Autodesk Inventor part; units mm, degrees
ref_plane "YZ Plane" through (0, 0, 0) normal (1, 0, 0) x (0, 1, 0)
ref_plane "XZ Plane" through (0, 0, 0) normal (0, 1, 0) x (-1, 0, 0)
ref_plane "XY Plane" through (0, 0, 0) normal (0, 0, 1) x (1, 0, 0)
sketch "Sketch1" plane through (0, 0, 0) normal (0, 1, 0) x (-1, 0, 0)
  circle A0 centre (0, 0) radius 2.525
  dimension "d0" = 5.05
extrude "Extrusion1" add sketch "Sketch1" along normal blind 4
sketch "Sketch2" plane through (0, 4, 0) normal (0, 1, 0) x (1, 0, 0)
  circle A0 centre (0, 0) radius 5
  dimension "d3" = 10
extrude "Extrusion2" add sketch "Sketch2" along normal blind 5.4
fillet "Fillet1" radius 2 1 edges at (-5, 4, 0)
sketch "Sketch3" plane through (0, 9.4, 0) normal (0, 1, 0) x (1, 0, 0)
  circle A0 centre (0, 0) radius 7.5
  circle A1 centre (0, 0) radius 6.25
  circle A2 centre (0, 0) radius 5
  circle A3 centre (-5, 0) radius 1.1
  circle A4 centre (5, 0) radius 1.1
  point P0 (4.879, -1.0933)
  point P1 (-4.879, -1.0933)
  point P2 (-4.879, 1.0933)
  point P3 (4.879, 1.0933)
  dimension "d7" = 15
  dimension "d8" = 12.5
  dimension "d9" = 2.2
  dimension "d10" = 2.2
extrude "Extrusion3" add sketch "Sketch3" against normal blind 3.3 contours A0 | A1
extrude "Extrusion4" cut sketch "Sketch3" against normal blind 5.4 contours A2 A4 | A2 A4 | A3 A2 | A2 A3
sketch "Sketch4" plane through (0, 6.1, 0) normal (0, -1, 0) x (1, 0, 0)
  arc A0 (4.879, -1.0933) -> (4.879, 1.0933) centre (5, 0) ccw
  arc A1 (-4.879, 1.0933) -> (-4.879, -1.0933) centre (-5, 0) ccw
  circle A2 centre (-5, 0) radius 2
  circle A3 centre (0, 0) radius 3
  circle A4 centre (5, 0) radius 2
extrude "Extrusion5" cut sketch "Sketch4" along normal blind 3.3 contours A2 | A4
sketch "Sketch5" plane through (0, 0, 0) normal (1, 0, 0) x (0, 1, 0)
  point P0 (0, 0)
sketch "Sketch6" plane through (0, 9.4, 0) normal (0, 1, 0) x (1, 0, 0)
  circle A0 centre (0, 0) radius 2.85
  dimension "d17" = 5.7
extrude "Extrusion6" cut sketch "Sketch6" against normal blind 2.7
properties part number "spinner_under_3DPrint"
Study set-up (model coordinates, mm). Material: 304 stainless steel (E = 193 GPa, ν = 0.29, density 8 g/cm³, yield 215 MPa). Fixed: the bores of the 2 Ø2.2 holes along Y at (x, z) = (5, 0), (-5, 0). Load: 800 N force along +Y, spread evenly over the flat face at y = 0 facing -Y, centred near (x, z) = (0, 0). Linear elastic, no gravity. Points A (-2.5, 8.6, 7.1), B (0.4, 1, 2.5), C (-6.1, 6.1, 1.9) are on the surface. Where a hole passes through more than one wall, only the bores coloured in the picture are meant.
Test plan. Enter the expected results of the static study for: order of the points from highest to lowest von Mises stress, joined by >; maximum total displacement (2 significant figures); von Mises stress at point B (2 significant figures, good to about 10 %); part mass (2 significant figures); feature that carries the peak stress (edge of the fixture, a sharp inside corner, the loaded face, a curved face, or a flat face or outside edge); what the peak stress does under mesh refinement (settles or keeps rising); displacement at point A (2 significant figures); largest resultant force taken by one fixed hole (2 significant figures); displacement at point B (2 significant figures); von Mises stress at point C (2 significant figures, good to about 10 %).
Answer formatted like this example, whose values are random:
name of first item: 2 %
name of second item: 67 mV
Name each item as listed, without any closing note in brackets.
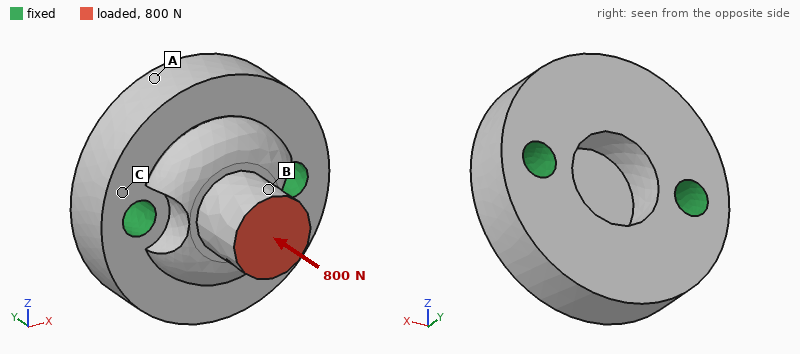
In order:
order of the points from highest to lowest von Mises stress, joined by >: B > C > A
maximum total displacement: 2.2 µm
von Mises stress at point B: 39 MPa
part mass: 5.5 g
feature that carries the peak stress: edge of the fixture
what the peak stress does under mesh refinement: keeps rising
displacement at point A: 1.1 µm
largest resultant force taken by one fixed hole: 430 N
displacement at point B: 2.0 µm
von Mises stress at point C: 14 MPa
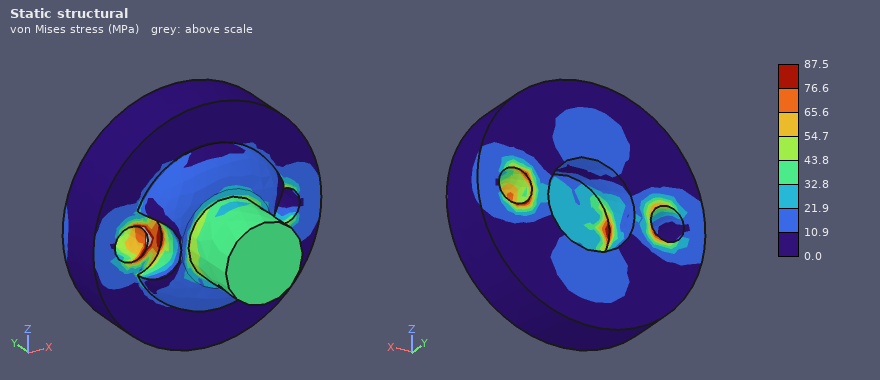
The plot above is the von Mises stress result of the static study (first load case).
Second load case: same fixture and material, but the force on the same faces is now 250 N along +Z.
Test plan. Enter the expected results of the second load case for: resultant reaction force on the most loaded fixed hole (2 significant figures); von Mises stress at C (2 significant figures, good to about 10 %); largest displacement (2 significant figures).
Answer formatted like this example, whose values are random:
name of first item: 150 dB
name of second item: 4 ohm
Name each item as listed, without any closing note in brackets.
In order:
resultant reaction force on the most loaded fixed hole: 130 N
von Mises stress at C: 25 MPa
largest displacement: 5.8 µm
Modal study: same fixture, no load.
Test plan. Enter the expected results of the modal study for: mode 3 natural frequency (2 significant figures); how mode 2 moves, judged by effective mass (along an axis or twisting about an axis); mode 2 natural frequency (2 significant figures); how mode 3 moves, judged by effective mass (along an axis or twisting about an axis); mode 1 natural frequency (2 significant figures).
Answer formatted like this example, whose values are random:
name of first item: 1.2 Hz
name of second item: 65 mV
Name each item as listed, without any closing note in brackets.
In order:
mode 3 natural frequency: 74 kHz
how mode 2 moves, judged by effective mass: along Y
mode 2 natural frequency: 60 kHz
how mode 3 moves, judged by effective mass: along X
mode 1 natural frequency: 38 kHz
